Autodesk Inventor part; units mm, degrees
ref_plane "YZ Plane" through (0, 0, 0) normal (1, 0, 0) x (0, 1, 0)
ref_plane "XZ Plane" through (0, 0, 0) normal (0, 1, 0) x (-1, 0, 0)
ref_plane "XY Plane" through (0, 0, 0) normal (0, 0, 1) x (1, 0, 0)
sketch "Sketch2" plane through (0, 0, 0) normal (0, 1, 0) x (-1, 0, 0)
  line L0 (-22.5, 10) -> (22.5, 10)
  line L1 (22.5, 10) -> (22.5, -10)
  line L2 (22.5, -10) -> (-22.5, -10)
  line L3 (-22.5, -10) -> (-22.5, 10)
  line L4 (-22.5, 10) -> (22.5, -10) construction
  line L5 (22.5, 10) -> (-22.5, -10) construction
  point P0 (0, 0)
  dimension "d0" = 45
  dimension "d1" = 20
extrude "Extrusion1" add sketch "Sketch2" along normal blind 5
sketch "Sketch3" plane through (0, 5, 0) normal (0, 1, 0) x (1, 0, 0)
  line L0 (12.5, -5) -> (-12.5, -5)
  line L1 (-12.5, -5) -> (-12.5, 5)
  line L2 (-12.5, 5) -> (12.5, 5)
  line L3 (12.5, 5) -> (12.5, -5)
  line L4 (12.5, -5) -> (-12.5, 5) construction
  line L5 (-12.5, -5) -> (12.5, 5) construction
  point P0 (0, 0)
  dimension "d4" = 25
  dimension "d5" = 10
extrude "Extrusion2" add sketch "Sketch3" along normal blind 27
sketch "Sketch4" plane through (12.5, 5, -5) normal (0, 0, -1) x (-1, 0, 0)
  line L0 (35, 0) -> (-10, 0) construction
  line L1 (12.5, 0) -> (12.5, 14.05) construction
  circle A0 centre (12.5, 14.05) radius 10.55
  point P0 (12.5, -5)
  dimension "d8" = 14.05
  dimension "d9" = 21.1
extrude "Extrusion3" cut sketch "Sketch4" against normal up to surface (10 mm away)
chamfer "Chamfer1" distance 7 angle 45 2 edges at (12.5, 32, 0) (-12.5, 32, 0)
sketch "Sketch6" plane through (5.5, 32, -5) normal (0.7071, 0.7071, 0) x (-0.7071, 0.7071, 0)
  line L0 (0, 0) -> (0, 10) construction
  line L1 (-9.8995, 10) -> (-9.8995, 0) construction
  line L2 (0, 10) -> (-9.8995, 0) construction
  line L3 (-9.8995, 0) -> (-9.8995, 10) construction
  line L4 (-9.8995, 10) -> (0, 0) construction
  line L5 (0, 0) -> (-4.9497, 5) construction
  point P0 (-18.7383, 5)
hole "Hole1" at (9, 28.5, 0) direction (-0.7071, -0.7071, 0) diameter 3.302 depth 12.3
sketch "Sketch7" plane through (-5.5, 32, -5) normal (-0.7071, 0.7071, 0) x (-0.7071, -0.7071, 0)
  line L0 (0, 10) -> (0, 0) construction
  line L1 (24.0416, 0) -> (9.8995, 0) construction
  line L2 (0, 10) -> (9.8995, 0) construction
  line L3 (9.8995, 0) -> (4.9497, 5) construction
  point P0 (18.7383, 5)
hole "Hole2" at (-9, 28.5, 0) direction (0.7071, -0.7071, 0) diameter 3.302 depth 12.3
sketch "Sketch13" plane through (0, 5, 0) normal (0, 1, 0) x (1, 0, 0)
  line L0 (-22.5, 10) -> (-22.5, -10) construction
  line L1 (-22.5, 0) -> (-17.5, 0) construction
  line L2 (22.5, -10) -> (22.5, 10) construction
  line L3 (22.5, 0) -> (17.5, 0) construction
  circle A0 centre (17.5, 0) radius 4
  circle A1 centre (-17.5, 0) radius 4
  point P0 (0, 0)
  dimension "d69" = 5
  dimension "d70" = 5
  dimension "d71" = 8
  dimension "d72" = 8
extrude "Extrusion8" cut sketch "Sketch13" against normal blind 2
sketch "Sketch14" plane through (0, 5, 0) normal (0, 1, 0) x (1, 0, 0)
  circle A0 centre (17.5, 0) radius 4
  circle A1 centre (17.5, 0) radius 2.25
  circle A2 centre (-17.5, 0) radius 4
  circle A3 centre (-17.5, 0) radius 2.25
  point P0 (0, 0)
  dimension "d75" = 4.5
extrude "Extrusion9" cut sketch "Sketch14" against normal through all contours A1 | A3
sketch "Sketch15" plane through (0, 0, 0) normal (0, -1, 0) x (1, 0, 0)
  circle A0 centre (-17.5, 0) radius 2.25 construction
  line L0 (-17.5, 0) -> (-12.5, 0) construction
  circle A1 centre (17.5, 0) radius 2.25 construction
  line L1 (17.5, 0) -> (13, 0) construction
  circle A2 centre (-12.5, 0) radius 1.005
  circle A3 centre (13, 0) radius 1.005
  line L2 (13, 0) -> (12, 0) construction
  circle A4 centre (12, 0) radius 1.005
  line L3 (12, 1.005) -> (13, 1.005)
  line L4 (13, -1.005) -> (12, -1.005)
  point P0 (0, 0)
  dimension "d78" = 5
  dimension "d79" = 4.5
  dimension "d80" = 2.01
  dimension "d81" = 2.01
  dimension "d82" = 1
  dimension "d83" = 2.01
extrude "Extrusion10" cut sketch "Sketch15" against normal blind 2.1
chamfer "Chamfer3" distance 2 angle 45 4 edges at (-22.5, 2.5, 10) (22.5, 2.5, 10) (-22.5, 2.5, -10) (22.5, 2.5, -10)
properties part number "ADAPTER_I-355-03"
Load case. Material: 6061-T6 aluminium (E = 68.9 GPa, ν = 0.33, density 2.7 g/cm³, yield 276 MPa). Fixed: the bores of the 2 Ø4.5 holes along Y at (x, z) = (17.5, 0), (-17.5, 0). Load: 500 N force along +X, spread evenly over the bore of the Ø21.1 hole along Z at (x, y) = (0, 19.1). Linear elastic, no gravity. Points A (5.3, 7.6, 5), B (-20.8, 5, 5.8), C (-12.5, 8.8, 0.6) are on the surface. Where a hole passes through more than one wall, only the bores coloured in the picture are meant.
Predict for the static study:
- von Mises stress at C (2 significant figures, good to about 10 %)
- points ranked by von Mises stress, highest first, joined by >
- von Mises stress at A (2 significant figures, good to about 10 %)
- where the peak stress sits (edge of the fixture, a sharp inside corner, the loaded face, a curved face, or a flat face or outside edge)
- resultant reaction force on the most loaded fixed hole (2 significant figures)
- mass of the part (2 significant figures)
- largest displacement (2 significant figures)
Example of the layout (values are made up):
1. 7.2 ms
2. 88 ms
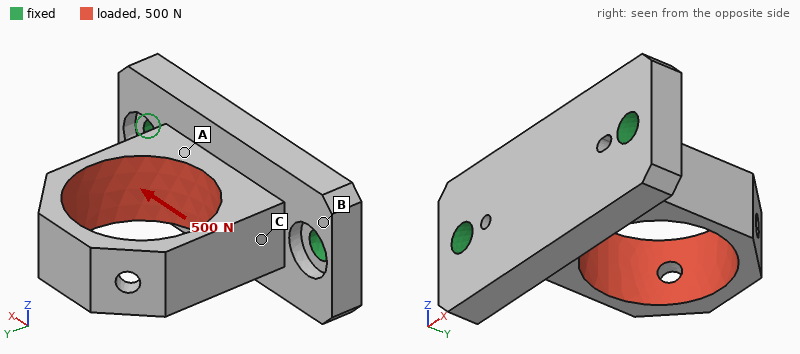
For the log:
1. 28 MPa
2. C > A > B
3. 12 MPa
4. the loaded face
5. 380 N
6. 19 g
7. 58 µm
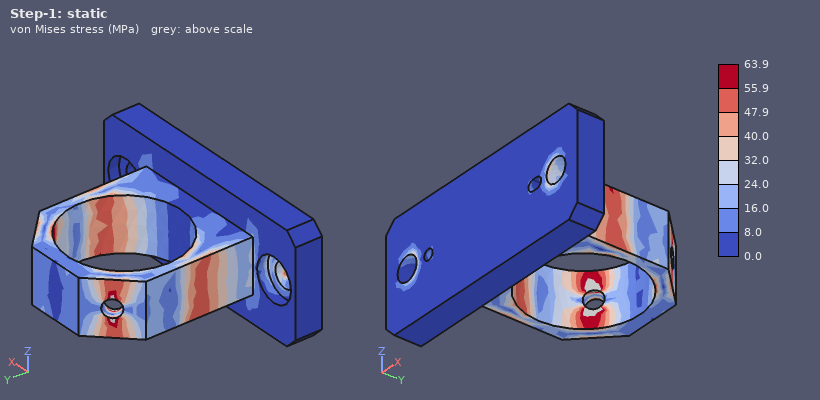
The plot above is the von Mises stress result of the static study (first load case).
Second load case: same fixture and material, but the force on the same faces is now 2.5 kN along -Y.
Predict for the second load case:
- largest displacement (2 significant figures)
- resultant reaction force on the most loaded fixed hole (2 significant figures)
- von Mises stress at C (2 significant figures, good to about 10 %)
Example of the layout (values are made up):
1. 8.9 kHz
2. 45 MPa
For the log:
1. 50 µm
2. 1.4 kN
3. 53 MPa
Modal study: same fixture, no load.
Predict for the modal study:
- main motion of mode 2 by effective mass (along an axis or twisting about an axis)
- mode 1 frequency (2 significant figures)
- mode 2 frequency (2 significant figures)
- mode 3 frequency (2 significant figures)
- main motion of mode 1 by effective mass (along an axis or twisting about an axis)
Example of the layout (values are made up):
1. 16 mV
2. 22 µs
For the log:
1. along X
2. 5000 Hz
3. 6900 Hz
4. 14 kHz
5. along Z
